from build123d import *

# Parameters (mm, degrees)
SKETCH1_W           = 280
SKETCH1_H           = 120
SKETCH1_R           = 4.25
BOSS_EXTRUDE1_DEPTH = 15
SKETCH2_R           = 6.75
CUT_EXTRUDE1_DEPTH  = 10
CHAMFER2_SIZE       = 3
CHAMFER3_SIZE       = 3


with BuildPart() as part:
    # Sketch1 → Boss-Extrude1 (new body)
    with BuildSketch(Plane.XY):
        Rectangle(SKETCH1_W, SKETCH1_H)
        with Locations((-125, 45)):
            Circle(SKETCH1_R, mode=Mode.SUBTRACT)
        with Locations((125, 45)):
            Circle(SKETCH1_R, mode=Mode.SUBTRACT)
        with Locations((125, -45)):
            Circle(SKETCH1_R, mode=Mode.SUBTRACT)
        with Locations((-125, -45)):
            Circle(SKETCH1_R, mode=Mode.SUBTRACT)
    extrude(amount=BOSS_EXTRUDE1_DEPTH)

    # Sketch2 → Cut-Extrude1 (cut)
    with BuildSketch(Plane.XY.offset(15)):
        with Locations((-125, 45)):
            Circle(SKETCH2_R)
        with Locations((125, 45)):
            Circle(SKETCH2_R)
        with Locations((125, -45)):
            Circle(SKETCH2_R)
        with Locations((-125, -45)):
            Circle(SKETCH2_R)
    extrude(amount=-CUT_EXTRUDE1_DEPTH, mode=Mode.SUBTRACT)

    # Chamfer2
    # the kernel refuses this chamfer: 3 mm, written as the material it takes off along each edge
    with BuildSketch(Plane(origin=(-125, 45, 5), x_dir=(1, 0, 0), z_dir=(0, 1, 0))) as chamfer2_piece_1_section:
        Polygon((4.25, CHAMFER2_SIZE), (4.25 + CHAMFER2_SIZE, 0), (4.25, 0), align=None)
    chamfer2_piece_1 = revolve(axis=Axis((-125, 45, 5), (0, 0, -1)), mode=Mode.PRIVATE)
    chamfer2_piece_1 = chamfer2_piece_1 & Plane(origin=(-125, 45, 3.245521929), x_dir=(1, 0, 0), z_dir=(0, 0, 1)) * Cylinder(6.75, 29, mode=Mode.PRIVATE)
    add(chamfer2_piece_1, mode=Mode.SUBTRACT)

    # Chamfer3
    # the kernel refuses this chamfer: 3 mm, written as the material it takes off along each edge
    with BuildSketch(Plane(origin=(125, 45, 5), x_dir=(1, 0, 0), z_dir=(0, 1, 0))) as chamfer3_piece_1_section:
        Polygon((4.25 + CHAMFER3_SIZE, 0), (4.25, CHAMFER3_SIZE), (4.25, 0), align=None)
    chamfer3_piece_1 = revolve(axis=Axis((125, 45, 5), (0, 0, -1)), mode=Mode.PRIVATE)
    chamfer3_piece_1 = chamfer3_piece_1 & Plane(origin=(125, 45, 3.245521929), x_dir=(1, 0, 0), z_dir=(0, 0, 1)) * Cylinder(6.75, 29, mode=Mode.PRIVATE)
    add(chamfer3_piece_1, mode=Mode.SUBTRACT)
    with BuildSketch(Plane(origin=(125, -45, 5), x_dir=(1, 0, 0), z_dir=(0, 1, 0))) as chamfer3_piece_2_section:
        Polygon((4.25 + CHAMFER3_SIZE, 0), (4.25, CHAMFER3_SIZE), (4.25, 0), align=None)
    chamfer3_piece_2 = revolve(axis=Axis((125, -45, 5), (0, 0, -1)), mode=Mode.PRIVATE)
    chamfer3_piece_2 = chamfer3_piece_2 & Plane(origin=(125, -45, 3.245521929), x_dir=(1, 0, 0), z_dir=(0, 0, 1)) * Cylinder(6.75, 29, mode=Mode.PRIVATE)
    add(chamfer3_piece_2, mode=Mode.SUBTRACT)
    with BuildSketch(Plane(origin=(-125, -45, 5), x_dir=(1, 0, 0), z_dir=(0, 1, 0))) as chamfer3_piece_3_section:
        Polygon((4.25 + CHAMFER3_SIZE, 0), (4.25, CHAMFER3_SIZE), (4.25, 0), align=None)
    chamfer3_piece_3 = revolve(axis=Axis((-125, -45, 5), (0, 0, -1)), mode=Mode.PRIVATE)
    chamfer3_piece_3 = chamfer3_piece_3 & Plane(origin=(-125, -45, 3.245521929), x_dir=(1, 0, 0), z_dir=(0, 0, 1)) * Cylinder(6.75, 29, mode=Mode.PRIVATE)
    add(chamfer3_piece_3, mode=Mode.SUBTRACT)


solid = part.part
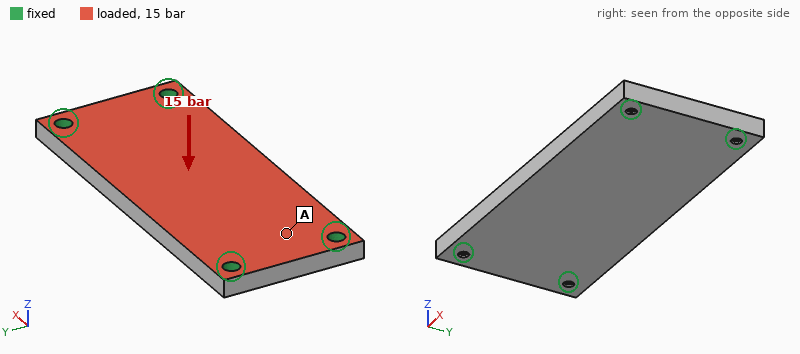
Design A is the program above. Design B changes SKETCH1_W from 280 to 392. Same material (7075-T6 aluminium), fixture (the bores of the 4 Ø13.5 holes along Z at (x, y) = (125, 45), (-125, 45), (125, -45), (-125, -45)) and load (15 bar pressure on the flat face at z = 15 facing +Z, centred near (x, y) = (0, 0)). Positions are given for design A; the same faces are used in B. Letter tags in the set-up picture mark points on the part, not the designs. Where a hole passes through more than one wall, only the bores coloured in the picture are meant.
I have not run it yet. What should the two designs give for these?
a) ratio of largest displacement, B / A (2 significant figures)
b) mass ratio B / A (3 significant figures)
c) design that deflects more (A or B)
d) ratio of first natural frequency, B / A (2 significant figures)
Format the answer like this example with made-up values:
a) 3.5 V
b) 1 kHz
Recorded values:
a) 0.89
b) 1.41
c) A
d) 1.0
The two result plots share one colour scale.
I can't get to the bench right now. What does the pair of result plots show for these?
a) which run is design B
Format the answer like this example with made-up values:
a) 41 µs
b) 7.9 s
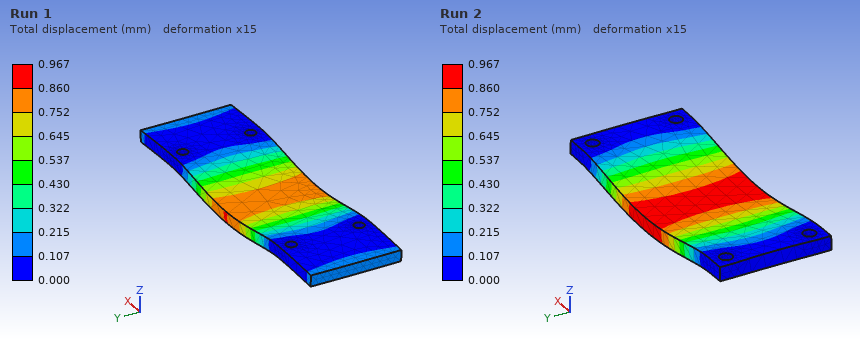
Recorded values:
a) Run 1
